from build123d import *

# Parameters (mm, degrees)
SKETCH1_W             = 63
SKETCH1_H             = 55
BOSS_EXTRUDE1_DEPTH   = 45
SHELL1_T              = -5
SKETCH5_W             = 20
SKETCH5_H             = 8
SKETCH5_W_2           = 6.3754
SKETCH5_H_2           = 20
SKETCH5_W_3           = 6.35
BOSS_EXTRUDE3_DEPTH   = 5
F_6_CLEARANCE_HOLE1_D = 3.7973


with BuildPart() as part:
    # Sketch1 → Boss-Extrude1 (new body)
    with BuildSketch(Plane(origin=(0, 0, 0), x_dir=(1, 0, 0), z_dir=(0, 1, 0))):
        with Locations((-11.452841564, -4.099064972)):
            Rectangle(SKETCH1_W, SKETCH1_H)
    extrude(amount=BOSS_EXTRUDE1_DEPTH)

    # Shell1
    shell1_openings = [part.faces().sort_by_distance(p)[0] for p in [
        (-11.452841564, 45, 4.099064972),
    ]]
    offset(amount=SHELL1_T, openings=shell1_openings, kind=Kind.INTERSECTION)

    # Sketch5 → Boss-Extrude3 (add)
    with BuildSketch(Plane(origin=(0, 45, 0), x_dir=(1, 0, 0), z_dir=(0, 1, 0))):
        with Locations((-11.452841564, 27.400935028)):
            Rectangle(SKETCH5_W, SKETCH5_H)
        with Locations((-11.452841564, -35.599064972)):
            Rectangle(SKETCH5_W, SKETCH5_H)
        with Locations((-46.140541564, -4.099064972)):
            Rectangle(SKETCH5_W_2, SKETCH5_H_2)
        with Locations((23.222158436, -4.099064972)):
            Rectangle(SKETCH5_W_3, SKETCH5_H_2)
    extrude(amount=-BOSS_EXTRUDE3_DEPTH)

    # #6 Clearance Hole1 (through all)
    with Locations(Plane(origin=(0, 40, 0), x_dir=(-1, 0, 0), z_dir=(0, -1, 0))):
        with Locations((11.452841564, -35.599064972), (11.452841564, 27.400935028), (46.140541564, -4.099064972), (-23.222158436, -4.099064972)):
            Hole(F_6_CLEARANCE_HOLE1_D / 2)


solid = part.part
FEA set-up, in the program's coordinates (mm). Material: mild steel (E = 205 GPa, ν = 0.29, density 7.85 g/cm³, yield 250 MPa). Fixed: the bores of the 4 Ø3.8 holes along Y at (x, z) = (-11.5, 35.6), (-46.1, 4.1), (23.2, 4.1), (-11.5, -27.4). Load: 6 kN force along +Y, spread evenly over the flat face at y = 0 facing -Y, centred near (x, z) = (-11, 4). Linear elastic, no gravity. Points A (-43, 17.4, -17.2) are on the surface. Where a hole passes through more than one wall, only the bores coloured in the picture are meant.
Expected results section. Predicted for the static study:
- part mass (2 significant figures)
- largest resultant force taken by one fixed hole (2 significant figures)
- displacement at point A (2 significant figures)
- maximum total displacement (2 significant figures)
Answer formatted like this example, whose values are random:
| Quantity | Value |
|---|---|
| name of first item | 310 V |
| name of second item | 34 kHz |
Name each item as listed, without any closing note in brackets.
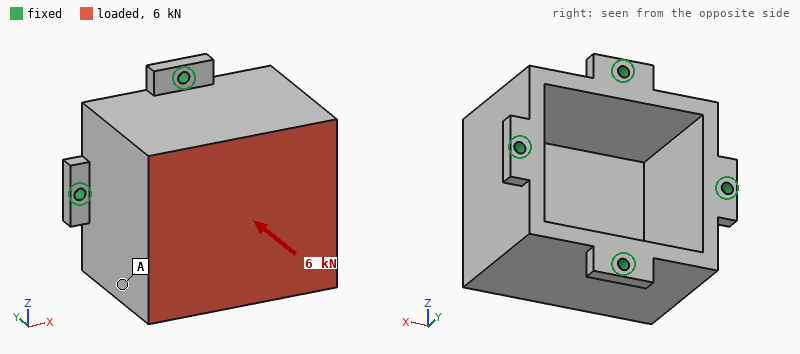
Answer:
| Quantity | Value |
|---|---|
| part mass | 500 g |
| largest resultant force taken by one fixed hole | 1.6 kN |
| displacement at point A | 4.2 µm |
| maximum total displacement | 17 µm |
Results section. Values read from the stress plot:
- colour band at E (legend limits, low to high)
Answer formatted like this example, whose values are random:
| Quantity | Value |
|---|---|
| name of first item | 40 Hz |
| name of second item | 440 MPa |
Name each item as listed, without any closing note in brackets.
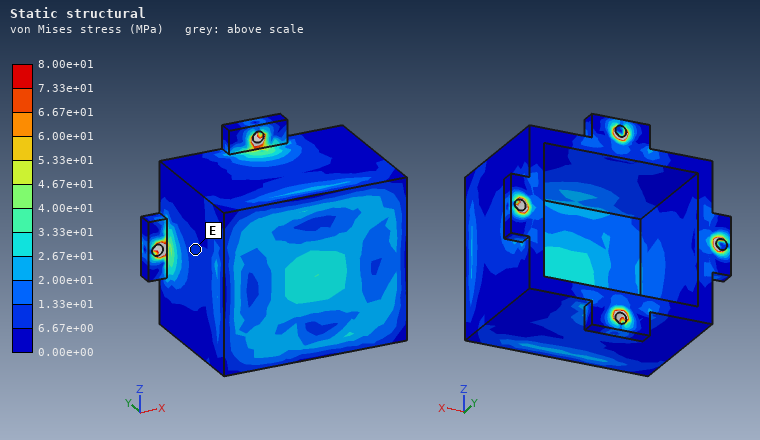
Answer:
| Quantity | Value |
|---|---|
| colour band at E | 6.67e+00 to 1.33e+01 MPa |
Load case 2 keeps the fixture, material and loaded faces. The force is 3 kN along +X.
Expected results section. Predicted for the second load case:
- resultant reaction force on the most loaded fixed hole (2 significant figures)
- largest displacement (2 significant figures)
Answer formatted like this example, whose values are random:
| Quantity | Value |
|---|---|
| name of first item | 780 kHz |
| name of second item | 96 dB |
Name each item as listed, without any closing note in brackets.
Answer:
| Quantity | Value |
|---|---|
| resultant reaction force on the most loaded fixed hole | 2.0 kN |
| largest displacement | 14 µm |
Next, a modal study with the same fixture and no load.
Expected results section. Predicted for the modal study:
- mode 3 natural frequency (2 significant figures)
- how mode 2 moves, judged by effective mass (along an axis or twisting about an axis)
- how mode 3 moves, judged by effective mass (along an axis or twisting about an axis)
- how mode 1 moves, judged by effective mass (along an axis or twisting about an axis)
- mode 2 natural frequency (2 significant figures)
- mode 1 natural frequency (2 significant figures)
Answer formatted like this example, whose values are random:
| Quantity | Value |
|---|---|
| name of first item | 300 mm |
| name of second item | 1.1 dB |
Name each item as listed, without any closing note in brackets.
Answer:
| Quantity | Value |
|---|---|
| mode 3 natural frequency | 8300 Hz |
| how mode 2 moves, judged by effective mass | along X |
| how mode 3 moves, judged by effective mass | along Y |
| how mode 1 moves, judged by effective mass | along Z |
| mode 2 natural frequency | 4800 Hz |
| mode 1 natural frequency | 4300 Hz |
